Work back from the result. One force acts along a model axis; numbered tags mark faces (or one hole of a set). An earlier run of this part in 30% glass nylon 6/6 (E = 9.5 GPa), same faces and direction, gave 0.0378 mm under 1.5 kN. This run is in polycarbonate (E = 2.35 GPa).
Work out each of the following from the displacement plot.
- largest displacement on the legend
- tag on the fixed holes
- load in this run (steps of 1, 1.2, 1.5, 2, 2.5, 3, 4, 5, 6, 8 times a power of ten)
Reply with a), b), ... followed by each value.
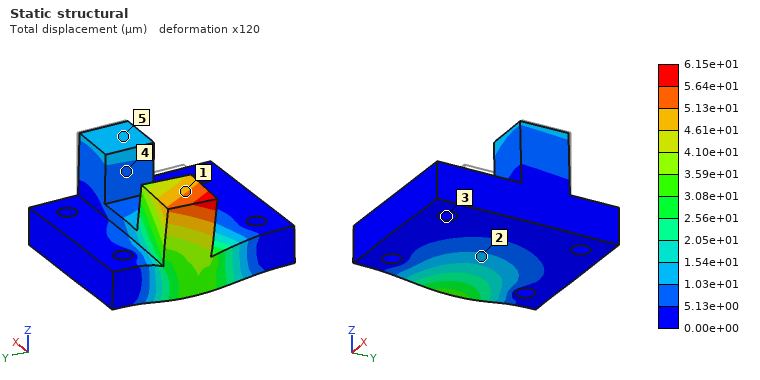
a) 6.15e+01 µm
b) 3
c) 600 N
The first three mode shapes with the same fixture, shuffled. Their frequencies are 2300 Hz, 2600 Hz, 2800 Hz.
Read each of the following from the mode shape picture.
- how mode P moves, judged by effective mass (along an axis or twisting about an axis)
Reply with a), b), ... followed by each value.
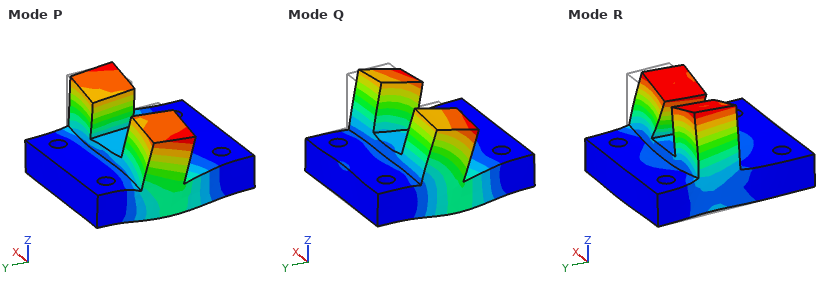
a) along X
